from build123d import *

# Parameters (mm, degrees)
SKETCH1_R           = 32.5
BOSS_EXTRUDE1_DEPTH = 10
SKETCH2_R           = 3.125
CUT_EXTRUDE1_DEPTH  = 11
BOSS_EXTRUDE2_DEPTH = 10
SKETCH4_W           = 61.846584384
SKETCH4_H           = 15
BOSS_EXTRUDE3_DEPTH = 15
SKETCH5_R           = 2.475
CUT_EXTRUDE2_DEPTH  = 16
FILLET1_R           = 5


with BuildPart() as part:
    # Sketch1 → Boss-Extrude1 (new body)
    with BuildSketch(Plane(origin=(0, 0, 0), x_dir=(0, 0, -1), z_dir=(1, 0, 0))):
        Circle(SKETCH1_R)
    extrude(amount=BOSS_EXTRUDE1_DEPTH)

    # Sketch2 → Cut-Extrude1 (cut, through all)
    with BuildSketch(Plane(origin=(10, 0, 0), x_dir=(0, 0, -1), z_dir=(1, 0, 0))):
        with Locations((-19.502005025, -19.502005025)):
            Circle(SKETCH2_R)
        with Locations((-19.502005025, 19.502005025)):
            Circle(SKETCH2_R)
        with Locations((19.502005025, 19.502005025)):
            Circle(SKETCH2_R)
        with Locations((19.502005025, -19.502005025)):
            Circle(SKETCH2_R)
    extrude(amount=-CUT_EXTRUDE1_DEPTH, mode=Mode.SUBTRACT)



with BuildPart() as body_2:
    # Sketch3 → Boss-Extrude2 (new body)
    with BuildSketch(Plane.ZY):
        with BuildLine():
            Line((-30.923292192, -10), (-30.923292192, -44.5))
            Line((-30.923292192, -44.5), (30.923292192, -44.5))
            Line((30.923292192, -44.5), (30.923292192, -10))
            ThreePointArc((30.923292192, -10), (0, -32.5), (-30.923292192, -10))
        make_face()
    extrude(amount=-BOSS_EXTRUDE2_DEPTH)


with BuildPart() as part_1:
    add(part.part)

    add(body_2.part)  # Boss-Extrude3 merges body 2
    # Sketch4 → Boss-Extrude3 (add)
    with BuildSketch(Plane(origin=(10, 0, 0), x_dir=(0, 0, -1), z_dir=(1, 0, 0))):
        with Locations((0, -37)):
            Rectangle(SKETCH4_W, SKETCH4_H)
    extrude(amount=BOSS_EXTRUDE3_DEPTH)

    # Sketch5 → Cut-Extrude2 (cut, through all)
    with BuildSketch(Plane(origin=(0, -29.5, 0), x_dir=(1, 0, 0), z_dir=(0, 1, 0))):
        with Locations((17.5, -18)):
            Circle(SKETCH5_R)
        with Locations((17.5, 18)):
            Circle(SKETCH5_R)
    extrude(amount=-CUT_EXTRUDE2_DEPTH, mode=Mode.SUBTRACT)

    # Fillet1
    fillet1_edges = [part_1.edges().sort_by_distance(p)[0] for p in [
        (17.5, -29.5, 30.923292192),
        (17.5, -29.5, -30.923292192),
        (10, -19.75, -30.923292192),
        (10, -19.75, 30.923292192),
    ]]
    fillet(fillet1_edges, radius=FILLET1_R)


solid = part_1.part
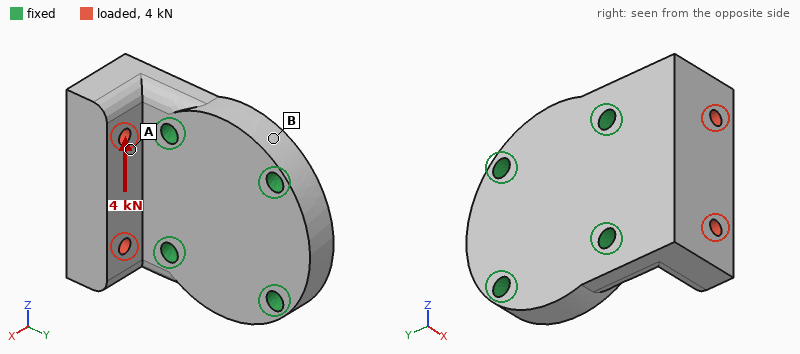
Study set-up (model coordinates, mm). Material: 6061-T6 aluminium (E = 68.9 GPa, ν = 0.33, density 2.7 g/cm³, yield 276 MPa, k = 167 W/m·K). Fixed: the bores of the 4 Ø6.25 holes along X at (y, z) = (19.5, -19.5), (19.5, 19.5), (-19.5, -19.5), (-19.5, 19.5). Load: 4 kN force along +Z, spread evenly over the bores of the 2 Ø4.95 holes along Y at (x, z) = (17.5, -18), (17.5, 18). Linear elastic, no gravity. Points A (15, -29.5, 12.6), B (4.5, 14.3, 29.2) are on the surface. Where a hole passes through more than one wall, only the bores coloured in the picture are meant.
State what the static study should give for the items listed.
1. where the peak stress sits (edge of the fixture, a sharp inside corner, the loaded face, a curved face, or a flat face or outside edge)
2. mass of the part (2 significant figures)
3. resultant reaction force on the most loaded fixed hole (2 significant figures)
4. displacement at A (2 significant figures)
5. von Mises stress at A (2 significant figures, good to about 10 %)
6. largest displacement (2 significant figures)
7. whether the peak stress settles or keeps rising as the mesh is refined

edge of the fixture
150 g
2.7 kN
9.5 µm
17 MPa
19 µm
keeps rising
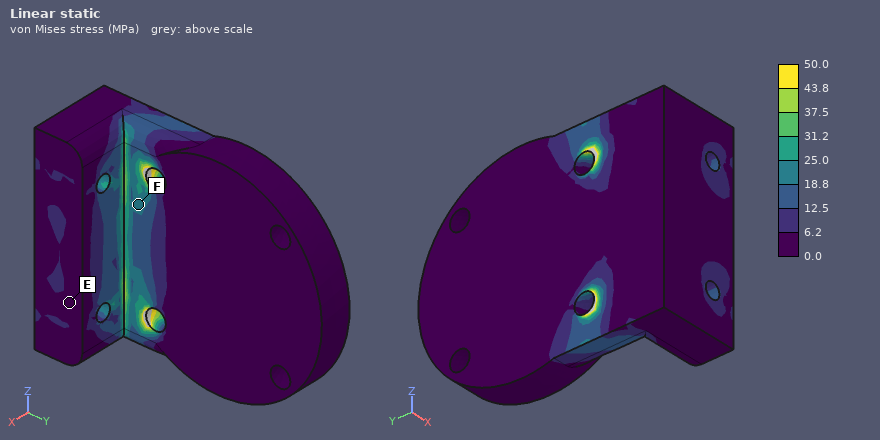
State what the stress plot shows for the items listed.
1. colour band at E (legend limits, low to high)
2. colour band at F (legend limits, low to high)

0.0 to 6.2 MPa
18.8 to 25.0 MPa
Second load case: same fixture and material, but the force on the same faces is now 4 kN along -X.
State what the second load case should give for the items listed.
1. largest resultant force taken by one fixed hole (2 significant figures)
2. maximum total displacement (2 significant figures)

2.2 kN
58 µm
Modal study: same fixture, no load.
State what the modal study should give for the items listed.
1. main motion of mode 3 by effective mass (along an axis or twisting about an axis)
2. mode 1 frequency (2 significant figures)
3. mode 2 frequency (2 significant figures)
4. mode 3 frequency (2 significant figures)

along Z
6000 Hz
11 kHz
16 kHz
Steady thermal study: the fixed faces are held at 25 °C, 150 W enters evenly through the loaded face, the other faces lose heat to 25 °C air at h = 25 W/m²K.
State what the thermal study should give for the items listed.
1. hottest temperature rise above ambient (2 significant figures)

40 K
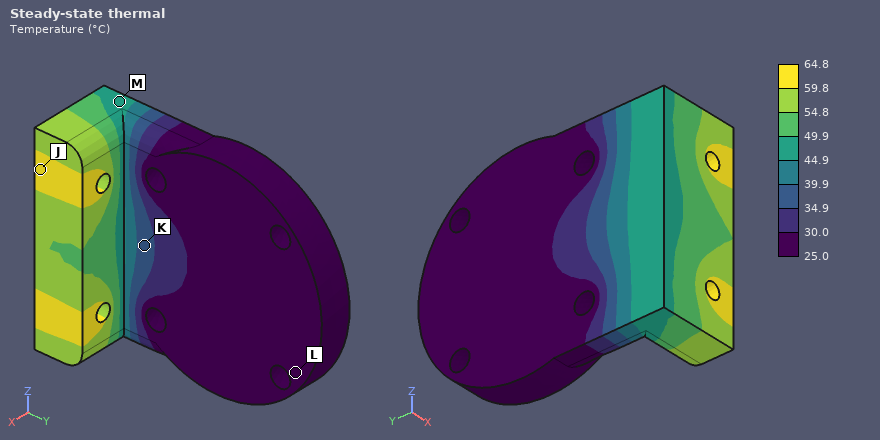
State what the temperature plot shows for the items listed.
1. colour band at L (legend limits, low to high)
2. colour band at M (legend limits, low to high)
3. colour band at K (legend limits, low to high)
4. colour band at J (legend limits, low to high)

25.0 to 30.0 °C
44.9 to 49.9 °C
34.9 to 39.9 °C
59.8 to 64.8 °C
